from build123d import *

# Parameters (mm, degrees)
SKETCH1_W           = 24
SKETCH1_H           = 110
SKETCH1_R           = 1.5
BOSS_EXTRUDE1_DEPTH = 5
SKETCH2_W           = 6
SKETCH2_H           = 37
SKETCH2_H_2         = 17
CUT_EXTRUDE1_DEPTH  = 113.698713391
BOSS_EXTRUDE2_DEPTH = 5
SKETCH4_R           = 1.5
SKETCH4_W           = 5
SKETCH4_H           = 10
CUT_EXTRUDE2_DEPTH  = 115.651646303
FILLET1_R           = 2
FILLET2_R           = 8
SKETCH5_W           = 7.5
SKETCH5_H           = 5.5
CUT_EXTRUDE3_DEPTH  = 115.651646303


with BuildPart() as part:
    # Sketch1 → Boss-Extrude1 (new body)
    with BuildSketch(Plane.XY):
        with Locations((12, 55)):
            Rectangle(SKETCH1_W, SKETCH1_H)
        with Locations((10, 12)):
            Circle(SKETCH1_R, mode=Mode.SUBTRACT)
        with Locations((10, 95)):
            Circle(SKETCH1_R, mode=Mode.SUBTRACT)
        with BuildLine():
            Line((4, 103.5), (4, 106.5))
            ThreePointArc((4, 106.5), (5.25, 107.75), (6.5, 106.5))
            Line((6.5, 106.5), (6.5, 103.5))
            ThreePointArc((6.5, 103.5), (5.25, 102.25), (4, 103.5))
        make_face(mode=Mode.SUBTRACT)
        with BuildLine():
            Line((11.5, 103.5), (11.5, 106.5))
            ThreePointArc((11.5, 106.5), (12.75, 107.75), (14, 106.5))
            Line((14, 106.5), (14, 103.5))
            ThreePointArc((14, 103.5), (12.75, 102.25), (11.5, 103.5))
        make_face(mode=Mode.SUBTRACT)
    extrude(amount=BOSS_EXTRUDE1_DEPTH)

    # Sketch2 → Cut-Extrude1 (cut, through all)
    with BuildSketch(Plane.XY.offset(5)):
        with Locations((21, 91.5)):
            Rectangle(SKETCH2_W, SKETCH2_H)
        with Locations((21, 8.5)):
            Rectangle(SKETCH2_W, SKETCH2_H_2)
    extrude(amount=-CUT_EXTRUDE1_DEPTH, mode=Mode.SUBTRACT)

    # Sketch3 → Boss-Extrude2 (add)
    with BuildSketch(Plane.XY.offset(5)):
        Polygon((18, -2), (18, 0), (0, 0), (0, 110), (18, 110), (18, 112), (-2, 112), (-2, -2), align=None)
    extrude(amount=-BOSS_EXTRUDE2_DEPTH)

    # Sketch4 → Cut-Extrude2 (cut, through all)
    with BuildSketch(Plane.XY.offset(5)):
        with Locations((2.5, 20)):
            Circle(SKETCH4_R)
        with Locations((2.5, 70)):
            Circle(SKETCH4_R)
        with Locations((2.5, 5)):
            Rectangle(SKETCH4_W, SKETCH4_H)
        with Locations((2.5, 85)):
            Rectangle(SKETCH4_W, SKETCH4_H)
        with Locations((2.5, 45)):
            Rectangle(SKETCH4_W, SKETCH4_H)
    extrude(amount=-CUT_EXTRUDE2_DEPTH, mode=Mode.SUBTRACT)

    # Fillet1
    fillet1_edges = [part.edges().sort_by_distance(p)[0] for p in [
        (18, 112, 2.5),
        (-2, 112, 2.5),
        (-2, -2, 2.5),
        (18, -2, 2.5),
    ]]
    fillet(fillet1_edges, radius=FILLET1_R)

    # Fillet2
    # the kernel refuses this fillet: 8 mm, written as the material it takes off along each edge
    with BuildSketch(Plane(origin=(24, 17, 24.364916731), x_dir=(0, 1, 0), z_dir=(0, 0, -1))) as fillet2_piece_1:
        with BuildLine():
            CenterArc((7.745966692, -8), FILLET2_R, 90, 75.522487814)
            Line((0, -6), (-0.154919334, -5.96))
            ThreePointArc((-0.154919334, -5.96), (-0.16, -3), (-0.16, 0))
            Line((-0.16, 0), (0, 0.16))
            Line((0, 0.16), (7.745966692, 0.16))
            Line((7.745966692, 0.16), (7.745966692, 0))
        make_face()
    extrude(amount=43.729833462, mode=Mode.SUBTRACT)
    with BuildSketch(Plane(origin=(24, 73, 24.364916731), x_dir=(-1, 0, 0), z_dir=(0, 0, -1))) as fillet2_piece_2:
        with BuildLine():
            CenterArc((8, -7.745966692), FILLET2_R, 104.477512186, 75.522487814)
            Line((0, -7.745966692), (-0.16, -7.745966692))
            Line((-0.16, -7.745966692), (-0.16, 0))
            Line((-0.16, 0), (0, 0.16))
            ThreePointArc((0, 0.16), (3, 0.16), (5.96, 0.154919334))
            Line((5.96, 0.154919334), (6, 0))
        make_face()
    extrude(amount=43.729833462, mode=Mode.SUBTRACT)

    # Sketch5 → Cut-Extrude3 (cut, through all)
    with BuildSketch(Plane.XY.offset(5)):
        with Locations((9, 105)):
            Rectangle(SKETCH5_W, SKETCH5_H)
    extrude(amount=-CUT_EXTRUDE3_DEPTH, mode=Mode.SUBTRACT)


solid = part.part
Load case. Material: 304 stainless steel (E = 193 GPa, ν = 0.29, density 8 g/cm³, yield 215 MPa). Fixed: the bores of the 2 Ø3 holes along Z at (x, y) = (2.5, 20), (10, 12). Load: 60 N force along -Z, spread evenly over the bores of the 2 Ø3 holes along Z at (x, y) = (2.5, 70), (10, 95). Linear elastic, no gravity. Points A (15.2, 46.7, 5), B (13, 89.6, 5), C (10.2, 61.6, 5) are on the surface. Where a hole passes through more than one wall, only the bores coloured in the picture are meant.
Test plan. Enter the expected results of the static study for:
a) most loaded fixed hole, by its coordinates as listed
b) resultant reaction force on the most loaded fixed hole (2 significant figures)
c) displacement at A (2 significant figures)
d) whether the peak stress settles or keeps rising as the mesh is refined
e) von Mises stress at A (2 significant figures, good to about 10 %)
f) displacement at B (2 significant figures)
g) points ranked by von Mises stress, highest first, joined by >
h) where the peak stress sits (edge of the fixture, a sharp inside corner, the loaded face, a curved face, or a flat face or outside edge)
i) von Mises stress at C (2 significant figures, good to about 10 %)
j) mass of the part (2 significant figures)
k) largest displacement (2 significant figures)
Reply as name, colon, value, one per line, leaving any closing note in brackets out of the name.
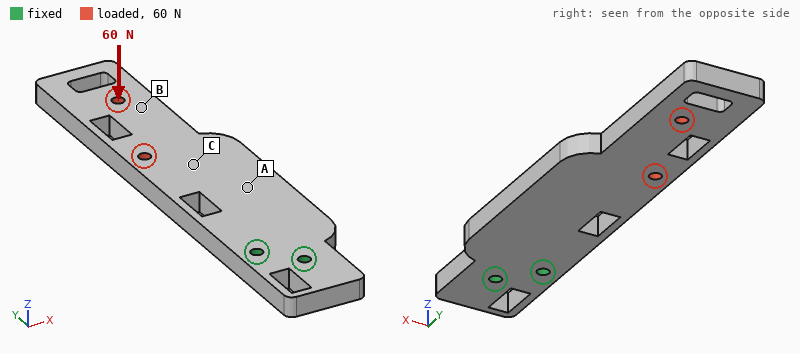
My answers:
most loaded fixed hole, by its coordinates as listed: (2.5, 20)
resultant reaction force on the most loaded fixed hole: 190 N
displacement at A: 0.030 mm
whether the peak stress settles or keeps rising as the mesh is refined: keeps rising
von Mises stress at A: 23 MPa
displacement at B: 0.14 mm
points ranked by von Mises stress, highest first, joined by >: A > C > B
where the peak stress sits: edge of the fixture
von Mises stress at C: 12 MPa
mass of the part: 94 g
largest displacement: 0.20 mm
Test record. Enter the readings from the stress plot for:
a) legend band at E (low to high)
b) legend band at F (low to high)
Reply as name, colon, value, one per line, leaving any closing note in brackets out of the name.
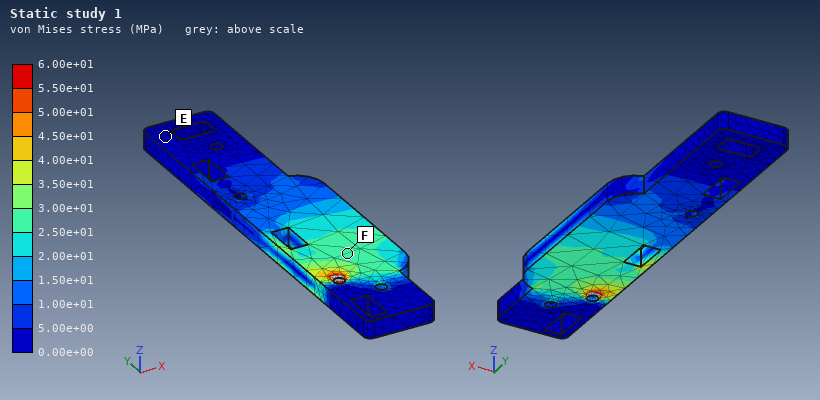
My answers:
legend band at E: 0.00e+00 to 5.00e+00 MPa
legend band at F: 2.50e+01 to 3.00e+01 MPa
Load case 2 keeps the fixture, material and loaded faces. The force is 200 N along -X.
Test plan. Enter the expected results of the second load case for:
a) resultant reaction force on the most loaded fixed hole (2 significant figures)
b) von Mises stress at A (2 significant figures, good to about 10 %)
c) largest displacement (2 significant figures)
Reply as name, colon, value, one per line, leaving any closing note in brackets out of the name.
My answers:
resultant reaction force on the most loaded fixed hole: 1.1 kN
von Mises stress at A: 6.3 MPa
largest displacement: 41 µm
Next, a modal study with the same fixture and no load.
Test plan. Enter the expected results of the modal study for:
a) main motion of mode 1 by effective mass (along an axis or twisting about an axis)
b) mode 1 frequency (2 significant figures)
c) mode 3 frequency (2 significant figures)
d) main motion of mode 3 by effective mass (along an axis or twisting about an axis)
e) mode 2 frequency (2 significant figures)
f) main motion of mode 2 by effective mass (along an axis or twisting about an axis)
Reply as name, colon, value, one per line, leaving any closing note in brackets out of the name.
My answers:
main motion of mode 1 by effective mass: along Z
mode 1 frequency: 510 Hz
mode 3 frequency: 2600 Hz
main motion of mode 3 by effective mass: along Z
mode 2 frequency: 2000 Hz
main motion of mode 2 by effective mass: along X
